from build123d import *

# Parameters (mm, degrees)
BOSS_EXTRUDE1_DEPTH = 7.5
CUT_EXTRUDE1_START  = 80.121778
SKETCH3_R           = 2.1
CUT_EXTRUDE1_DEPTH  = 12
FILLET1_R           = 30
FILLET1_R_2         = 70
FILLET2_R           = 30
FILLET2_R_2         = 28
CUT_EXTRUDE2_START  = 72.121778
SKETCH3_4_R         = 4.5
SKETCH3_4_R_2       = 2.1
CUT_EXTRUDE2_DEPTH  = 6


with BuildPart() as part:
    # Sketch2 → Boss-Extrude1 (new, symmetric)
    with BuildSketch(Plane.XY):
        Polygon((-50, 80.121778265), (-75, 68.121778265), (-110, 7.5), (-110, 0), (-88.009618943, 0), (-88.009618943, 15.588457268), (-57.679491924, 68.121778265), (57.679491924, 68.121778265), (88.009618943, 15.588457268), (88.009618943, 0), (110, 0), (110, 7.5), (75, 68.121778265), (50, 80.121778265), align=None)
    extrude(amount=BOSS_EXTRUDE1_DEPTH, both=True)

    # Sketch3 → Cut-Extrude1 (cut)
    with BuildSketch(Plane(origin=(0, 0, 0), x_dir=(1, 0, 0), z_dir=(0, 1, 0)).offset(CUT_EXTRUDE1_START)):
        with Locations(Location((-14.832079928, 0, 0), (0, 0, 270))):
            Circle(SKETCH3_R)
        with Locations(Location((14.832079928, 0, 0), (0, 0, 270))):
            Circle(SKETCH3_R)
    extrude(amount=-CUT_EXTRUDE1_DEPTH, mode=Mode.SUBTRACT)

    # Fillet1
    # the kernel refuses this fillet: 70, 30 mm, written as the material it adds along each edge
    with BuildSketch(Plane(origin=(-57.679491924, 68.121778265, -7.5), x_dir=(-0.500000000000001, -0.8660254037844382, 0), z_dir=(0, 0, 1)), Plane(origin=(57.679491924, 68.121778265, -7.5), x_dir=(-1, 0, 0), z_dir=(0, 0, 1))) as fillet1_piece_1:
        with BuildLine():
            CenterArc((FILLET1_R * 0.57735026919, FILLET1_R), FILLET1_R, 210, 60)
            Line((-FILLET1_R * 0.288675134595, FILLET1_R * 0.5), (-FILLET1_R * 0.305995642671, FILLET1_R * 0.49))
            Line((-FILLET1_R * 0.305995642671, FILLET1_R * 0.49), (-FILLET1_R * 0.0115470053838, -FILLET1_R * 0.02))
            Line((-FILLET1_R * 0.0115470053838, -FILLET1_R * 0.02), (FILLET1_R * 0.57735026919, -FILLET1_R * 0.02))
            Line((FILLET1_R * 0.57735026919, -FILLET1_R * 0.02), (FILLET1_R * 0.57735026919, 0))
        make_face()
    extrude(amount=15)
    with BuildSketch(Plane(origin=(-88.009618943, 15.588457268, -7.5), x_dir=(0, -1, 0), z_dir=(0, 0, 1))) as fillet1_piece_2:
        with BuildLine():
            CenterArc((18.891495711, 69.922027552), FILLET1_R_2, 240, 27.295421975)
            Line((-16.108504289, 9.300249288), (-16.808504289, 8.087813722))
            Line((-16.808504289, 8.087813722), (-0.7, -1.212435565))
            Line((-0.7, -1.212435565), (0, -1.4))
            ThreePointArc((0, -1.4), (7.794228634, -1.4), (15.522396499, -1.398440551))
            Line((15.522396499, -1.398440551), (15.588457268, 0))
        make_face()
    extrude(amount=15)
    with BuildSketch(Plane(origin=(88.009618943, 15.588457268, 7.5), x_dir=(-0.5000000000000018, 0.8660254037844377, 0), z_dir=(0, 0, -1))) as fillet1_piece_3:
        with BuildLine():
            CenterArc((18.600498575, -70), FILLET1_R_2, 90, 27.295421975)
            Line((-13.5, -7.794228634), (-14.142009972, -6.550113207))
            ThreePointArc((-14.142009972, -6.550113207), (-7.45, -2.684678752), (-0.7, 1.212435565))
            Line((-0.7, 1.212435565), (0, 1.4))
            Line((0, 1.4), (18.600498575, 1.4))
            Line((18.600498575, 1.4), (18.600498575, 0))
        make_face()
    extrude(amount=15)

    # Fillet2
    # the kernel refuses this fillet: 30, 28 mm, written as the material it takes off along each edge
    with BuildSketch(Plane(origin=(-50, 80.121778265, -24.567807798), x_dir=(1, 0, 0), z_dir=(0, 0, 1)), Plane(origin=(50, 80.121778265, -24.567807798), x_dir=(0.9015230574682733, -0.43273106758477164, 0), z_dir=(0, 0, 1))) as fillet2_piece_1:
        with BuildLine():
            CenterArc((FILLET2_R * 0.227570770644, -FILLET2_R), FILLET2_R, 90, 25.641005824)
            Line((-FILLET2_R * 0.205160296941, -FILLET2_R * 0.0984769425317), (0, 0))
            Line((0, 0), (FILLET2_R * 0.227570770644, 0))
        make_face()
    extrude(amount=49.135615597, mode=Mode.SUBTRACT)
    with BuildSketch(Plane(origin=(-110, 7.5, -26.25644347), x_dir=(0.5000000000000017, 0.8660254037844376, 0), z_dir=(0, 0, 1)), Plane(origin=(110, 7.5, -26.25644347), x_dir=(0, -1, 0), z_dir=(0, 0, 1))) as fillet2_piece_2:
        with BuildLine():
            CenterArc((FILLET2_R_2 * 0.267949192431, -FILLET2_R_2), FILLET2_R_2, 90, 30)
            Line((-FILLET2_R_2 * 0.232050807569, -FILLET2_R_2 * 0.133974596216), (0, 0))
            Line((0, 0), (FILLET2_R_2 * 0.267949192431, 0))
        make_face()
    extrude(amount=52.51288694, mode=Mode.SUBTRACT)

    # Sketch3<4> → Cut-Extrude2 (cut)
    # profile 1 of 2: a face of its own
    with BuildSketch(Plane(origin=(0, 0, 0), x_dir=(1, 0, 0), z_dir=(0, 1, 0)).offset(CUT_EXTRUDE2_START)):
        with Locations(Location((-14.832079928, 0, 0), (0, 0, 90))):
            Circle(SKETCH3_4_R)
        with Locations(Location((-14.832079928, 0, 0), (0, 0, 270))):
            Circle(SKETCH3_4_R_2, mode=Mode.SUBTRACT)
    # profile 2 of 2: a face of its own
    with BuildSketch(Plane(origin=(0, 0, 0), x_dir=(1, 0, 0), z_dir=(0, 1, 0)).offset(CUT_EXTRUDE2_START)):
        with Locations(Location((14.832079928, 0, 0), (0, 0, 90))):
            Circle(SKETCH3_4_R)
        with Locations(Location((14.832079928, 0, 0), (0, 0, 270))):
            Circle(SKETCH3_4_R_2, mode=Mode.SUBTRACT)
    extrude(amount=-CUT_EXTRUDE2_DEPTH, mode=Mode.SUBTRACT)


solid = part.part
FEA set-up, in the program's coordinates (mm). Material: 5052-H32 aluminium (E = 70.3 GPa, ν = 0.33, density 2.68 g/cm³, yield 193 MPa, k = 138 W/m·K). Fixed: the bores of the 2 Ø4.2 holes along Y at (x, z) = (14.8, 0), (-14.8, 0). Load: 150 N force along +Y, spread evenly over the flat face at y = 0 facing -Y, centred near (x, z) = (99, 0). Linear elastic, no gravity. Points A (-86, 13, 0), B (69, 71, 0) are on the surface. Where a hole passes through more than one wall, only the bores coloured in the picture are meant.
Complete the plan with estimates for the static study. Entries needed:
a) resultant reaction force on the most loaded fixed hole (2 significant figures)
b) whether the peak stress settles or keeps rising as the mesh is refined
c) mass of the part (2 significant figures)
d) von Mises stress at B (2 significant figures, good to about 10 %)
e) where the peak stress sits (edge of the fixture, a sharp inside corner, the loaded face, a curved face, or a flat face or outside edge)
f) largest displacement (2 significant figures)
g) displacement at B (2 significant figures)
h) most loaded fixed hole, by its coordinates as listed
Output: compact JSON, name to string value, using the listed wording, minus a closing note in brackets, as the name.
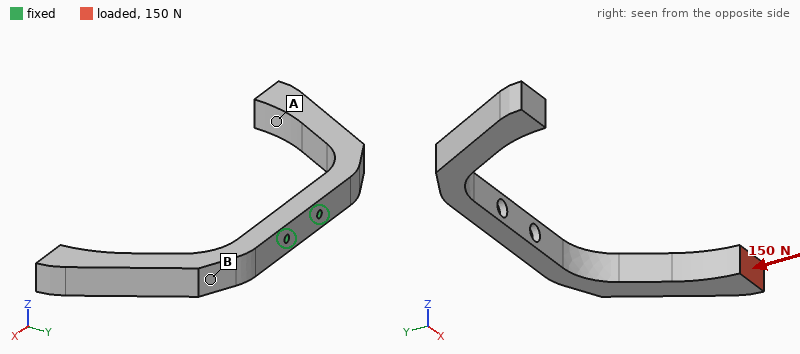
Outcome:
{"resultant reaction force on the most loaded fixed hole": "400 N", "whether the peak stress settles or keeps rising as the mesh is refined": "keeps rising", "mass of the part": "160 g", "von Mises stress at B": "10 MPa", "where the peak stress sits": "edge of the fixture", "largest displacement": "0.40 mm", "displacement at B": "0.13 mm", "most loaded fixed hole, by its coordinates as listed": "(14.8, 0)"}
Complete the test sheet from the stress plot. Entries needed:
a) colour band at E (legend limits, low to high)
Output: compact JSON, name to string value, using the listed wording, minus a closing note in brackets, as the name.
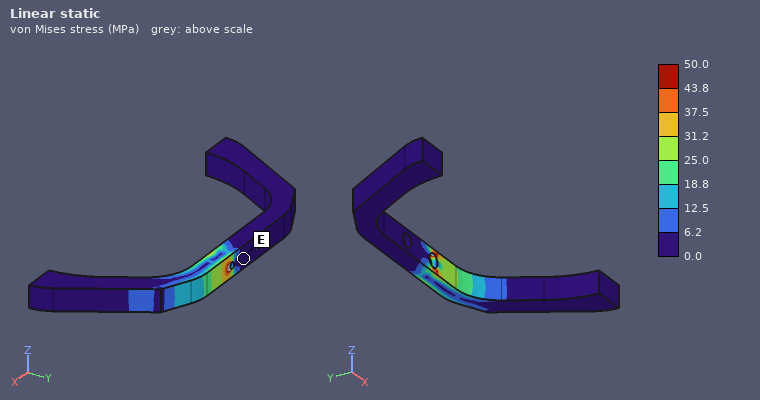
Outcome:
{"colour band at E": "0.0 to 6.2 MPa"}
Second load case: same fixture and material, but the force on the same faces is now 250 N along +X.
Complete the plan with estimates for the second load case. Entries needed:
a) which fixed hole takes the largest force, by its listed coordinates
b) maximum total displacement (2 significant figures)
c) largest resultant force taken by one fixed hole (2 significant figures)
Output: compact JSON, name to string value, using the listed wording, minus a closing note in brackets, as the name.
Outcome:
{"which fixed hole takes the largest force, by its listed coordinates": "(-14.8, 0)", "maximum total displacement": "0.82 mm", "largest resultant force taken by one fixed hole": "480 N"}
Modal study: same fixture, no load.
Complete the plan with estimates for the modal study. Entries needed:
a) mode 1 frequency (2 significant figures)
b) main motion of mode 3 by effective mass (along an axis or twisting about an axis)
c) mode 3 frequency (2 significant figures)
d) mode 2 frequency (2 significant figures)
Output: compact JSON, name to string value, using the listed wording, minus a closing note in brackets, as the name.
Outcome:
{"mode 1 frequency": "510 Hz", "main motion of mode 3 by effective mass": "along Z", "mode 3 frequency": "540 Hz", "mode 2 frequency": "510 Hz"}
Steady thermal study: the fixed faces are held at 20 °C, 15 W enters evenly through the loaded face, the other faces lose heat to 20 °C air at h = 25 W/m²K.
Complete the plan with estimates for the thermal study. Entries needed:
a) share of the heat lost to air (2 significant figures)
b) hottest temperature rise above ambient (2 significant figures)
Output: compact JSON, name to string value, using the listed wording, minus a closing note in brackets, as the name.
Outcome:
{"share of the heat lost to air": "34 %", "hottest temperature rise above ambient": "50 K"}
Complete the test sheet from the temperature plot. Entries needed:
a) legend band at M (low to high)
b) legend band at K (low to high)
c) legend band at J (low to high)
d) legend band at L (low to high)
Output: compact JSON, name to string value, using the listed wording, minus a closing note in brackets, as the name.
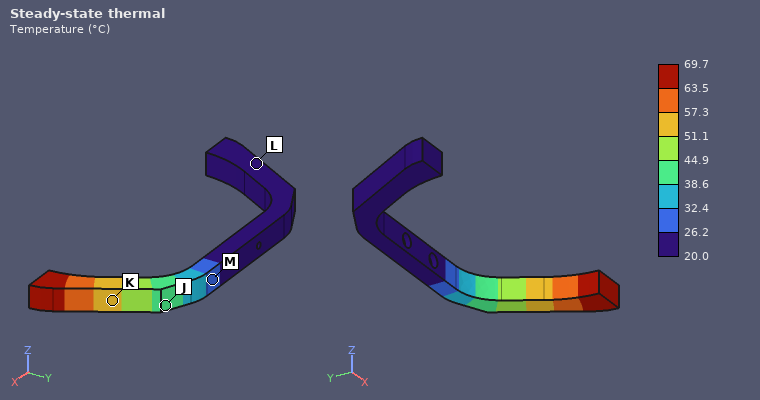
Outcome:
{"legend band at M": "26.2 to 32.4 °C", "legend band at K": "51.1 to 57.3 °C", "legend band at J": "38.6 to 44.9 °C", "legend band at L": "20.0 to 26.2 °C"}
